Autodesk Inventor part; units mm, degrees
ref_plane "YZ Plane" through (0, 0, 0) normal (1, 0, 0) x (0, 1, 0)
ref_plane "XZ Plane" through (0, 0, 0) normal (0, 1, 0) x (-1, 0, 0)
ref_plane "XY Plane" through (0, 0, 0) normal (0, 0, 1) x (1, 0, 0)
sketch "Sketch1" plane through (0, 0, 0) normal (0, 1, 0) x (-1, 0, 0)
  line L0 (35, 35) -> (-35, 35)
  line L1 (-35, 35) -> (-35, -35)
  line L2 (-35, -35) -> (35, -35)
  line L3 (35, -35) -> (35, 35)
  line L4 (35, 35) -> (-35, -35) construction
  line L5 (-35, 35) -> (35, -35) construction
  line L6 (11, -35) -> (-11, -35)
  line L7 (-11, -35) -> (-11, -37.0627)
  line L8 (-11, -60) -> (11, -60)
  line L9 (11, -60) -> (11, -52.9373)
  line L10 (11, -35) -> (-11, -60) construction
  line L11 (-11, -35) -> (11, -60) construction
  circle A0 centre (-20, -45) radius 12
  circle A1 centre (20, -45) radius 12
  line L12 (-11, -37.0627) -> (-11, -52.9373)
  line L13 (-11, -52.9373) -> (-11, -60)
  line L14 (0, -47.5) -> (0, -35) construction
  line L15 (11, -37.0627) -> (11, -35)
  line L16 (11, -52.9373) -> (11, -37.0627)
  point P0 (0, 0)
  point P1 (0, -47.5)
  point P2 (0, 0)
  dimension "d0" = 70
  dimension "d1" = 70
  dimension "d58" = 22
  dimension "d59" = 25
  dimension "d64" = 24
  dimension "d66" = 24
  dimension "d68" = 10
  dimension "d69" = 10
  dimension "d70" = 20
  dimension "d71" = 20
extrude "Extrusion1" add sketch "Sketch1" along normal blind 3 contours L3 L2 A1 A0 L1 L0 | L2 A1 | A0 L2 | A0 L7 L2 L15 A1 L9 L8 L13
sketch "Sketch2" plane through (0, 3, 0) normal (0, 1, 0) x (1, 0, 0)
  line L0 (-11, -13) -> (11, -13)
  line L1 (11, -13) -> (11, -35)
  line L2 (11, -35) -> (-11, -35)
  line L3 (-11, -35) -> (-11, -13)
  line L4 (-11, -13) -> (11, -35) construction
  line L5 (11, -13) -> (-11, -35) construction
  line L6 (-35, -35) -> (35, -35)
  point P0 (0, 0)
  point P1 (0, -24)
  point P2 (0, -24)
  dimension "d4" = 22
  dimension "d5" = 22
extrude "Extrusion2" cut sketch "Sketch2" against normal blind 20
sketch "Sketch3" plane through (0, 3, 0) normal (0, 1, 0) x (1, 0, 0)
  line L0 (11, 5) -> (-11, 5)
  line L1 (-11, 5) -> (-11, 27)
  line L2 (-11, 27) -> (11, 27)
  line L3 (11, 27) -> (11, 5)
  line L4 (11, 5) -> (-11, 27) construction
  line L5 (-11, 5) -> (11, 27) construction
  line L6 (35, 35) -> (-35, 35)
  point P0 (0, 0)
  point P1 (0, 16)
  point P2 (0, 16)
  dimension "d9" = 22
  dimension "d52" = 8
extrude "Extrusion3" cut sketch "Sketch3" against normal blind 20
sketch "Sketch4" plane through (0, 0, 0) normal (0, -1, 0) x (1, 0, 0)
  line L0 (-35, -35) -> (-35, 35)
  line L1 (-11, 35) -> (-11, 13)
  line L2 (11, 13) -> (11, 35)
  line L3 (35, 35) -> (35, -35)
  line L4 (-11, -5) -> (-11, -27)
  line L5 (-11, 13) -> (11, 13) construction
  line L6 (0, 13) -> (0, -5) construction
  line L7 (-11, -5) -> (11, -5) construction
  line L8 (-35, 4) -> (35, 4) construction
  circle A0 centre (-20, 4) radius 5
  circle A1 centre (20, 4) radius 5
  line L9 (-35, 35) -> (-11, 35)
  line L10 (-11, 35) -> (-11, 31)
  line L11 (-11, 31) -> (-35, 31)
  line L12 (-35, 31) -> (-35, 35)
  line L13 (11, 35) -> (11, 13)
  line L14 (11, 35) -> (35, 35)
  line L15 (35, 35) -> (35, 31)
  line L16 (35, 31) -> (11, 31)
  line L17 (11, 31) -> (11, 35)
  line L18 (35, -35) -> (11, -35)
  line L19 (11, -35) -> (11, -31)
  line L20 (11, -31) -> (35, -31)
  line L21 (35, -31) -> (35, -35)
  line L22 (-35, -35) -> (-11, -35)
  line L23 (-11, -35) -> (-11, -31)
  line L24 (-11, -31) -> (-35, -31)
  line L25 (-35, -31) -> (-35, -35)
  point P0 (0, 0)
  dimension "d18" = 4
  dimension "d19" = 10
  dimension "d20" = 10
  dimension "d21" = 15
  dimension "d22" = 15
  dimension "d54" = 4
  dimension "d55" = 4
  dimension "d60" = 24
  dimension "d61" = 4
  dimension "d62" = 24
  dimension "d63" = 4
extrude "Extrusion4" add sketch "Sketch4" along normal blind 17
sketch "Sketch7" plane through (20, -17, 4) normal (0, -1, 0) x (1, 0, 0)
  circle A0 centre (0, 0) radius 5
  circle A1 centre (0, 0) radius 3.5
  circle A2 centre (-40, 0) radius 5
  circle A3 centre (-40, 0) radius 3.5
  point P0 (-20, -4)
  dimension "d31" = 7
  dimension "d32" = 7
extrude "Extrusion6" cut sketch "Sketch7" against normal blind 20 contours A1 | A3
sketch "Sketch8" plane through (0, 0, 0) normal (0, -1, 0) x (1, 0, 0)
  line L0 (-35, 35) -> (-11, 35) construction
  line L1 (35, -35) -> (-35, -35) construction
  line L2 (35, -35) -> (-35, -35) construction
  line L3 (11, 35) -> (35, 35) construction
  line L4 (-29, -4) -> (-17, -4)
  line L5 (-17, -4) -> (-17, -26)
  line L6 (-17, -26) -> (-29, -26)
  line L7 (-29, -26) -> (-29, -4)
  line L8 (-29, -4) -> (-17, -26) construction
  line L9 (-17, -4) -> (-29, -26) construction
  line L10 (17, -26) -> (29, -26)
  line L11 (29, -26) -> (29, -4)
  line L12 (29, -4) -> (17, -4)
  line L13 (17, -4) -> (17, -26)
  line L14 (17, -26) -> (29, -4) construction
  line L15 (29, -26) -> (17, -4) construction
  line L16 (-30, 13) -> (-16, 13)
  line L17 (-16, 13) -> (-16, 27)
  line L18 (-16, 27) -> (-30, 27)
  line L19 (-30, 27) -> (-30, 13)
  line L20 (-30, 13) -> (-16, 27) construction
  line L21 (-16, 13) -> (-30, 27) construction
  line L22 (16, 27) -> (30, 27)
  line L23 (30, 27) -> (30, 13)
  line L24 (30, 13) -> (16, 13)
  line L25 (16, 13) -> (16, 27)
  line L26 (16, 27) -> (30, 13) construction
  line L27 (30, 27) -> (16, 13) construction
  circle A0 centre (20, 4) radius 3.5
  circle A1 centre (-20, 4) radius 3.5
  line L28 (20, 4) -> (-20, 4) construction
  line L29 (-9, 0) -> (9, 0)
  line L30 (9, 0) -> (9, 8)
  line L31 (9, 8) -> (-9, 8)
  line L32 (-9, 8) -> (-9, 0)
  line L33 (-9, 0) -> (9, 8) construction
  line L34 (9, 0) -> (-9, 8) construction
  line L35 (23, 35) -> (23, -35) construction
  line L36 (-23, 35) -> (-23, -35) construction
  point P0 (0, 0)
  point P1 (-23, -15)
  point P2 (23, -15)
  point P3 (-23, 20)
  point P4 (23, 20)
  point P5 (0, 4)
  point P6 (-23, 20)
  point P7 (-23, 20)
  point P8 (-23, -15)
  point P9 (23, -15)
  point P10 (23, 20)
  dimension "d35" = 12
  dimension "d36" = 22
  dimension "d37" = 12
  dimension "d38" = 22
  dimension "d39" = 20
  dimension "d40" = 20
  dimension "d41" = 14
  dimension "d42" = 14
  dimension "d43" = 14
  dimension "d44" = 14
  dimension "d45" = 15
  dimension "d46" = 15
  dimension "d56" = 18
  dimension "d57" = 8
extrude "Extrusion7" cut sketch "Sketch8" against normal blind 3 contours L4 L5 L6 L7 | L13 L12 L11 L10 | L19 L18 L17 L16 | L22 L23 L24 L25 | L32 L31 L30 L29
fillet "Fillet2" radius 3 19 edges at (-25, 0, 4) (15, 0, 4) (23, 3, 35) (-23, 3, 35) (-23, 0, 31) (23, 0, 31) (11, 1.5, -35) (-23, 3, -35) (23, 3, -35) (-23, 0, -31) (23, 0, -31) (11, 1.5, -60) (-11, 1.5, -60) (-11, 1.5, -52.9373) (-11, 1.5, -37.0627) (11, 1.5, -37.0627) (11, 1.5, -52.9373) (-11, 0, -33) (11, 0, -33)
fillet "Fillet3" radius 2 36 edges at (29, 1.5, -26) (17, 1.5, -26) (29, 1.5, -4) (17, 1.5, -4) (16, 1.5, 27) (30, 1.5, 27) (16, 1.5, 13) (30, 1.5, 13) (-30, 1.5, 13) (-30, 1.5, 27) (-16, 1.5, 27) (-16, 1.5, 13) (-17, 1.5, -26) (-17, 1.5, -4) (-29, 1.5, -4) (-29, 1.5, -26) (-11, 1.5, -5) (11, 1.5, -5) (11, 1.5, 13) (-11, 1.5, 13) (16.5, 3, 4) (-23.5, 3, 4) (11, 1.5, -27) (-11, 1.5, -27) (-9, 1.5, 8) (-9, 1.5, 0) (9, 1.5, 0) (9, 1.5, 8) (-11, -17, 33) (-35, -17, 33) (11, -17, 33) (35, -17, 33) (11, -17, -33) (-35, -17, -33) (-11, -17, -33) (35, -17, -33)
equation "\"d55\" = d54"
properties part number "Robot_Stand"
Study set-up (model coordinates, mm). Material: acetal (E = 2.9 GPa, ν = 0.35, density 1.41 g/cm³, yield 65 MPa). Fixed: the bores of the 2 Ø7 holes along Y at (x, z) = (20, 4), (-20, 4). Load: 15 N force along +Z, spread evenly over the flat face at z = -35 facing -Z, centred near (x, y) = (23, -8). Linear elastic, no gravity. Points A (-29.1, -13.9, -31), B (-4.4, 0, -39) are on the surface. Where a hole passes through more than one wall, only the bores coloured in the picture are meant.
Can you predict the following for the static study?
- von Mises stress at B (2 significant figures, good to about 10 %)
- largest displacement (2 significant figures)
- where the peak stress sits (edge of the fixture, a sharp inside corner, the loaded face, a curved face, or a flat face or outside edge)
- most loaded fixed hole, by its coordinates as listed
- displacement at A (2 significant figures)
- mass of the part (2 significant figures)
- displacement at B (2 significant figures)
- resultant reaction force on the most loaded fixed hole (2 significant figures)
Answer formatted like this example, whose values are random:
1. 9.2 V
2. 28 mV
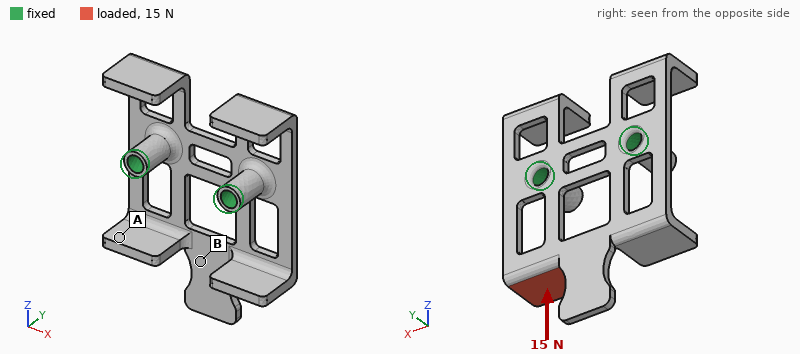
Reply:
1. 1.1 MPa
2. 1.3 mm
3. a curved face
4. (20, 4)
5. 0.46 mm
6. 25 g
7. 0.63 mm
8. 16 N
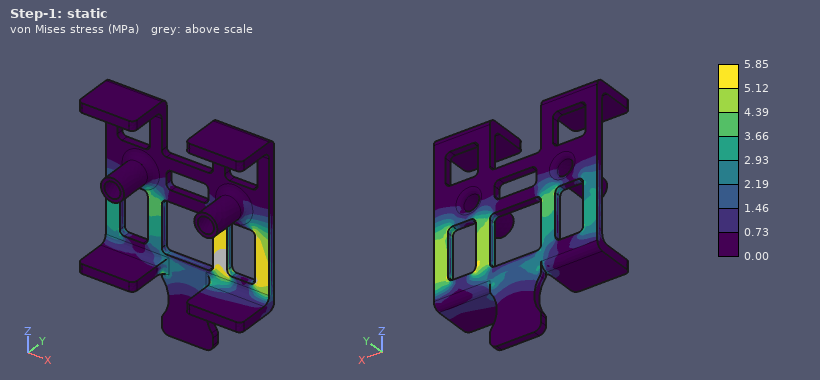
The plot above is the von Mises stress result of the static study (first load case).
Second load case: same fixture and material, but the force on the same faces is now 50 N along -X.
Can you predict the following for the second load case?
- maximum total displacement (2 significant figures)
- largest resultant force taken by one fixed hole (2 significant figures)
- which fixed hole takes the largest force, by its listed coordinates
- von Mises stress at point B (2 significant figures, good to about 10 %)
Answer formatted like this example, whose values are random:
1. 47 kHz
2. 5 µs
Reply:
1. 1.4 mm
2. 36 N
3. (20, 4)
4. 5.0 MPa
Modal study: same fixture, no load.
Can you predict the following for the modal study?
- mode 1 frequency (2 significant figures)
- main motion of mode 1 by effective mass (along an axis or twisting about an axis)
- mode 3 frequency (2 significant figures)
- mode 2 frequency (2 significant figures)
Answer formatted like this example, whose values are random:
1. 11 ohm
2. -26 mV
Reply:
1. 150 Hz
2. along Y
3. 290 Hz
4. 290 Hz
